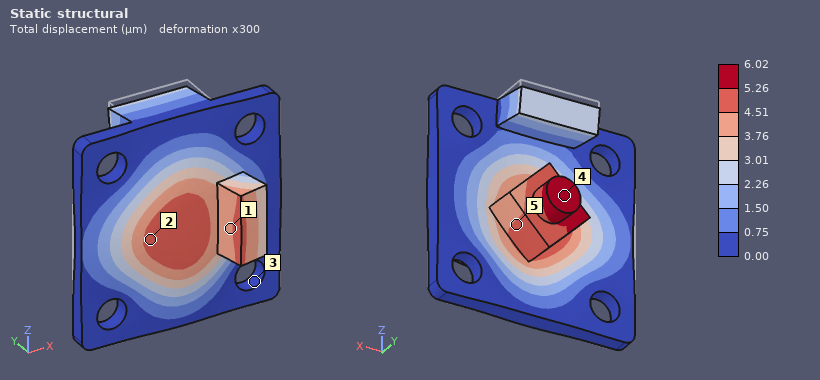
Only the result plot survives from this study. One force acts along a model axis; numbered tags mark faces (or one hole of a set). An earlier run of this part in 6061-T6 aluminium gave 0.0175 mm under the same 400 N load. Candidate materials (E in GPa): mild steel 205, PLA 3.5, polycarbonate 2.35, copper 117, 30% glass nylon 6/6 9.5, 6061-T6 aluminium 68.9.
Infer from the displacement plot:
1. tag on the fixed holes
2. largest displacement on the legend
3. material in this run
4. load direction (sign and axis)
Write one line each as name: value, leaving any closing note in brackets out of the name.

tag on the fixed holes: 3
largest displacement on the legend: 6.02 µm
material in this run: mild steel
load direction: -Y
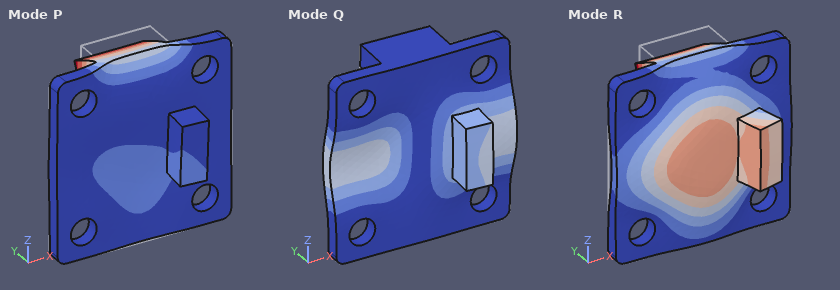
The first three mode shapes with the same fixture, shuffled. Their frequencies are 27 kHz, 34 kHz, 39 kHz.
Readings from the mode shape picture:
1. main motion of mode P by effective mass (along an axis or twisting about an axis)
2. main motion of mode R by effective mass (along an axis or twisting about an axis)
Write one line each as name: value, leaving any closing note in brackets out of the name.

main motion of mode P by effective mass: along Y
main motion of mode R by effective mass: along Y
